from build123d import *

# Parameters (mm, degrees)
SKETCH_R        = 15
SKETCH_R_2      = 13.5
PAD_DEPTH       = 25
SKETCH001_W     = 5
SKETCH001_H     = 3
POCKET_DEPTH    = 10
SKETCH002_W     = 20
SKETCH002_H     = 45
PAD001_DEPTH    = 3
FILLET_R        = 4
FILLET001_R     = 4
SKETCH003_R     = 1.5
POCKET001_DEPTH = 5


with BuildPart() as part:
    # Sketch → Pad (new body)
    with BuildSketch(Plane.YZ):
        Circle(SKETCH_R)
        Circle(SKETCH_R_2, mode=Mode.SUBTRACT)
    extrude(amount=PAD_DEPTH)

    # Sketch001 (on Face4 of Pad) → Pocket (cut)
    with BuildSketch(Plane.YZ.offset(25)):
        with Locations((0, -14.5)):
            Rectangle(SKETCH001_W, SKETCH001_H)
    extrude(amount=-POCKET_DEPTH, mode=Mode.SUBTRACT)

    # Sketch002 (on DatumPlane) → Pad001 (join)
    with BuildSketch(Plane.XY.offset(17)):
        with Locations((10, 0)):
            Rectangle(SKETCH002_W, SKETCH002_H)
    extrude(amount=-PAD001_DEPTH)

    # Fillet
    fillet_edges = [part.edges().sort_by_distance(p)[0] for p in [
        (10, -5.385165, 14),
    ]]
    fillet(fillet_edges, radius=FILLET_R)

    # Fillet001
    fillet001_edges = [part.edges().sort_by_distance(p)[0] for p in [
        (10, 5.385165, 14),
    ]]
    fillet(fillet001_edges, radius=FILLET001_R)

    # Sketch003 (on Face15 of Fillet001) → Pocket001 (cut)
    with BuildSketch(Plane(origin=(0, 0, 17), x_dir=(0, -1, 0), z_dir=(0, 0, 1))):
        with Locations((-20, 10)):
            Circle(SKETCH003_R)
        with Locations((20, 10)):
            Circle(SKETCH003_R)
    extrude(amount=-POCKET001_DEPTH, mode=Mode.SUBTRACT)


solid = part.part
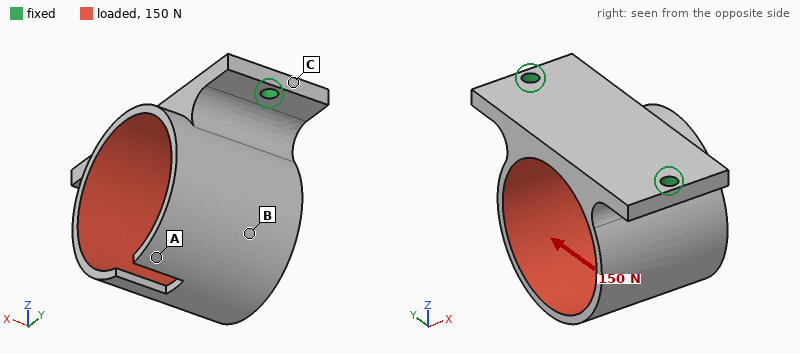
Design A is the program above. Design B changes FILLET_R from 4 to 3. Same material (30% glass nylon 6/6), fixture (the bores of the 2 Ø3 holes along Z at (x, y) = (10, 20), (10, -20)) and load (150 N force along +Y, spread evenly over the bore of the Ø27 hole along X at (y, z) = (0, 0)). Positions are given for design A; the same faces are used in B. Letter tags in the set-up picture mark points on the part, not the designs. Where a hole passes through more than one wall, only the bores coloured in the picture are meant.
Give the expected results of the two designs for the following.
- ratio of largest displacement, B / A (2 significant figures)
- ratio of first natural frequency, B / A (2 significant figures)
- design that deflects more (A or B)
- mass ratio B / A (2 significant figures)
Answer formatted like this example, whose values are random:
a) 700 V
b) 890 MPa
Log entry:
a) 1.1
b) 0.95
c) B
d) 0.98
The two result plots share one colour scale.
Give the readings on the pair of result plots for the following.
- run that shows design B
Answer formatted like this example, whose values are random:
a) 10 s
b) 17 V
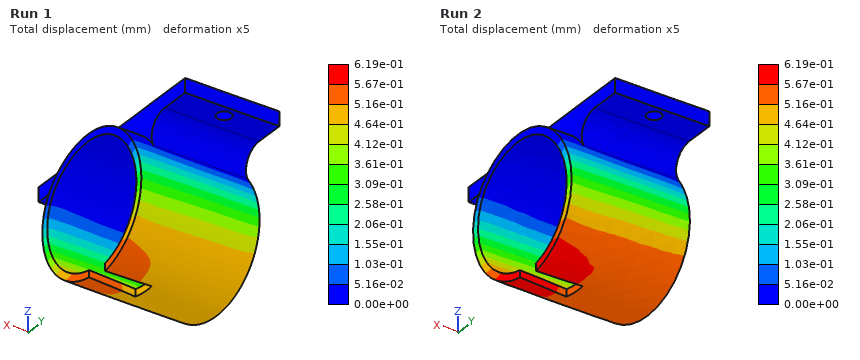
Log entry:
a) Run 2
